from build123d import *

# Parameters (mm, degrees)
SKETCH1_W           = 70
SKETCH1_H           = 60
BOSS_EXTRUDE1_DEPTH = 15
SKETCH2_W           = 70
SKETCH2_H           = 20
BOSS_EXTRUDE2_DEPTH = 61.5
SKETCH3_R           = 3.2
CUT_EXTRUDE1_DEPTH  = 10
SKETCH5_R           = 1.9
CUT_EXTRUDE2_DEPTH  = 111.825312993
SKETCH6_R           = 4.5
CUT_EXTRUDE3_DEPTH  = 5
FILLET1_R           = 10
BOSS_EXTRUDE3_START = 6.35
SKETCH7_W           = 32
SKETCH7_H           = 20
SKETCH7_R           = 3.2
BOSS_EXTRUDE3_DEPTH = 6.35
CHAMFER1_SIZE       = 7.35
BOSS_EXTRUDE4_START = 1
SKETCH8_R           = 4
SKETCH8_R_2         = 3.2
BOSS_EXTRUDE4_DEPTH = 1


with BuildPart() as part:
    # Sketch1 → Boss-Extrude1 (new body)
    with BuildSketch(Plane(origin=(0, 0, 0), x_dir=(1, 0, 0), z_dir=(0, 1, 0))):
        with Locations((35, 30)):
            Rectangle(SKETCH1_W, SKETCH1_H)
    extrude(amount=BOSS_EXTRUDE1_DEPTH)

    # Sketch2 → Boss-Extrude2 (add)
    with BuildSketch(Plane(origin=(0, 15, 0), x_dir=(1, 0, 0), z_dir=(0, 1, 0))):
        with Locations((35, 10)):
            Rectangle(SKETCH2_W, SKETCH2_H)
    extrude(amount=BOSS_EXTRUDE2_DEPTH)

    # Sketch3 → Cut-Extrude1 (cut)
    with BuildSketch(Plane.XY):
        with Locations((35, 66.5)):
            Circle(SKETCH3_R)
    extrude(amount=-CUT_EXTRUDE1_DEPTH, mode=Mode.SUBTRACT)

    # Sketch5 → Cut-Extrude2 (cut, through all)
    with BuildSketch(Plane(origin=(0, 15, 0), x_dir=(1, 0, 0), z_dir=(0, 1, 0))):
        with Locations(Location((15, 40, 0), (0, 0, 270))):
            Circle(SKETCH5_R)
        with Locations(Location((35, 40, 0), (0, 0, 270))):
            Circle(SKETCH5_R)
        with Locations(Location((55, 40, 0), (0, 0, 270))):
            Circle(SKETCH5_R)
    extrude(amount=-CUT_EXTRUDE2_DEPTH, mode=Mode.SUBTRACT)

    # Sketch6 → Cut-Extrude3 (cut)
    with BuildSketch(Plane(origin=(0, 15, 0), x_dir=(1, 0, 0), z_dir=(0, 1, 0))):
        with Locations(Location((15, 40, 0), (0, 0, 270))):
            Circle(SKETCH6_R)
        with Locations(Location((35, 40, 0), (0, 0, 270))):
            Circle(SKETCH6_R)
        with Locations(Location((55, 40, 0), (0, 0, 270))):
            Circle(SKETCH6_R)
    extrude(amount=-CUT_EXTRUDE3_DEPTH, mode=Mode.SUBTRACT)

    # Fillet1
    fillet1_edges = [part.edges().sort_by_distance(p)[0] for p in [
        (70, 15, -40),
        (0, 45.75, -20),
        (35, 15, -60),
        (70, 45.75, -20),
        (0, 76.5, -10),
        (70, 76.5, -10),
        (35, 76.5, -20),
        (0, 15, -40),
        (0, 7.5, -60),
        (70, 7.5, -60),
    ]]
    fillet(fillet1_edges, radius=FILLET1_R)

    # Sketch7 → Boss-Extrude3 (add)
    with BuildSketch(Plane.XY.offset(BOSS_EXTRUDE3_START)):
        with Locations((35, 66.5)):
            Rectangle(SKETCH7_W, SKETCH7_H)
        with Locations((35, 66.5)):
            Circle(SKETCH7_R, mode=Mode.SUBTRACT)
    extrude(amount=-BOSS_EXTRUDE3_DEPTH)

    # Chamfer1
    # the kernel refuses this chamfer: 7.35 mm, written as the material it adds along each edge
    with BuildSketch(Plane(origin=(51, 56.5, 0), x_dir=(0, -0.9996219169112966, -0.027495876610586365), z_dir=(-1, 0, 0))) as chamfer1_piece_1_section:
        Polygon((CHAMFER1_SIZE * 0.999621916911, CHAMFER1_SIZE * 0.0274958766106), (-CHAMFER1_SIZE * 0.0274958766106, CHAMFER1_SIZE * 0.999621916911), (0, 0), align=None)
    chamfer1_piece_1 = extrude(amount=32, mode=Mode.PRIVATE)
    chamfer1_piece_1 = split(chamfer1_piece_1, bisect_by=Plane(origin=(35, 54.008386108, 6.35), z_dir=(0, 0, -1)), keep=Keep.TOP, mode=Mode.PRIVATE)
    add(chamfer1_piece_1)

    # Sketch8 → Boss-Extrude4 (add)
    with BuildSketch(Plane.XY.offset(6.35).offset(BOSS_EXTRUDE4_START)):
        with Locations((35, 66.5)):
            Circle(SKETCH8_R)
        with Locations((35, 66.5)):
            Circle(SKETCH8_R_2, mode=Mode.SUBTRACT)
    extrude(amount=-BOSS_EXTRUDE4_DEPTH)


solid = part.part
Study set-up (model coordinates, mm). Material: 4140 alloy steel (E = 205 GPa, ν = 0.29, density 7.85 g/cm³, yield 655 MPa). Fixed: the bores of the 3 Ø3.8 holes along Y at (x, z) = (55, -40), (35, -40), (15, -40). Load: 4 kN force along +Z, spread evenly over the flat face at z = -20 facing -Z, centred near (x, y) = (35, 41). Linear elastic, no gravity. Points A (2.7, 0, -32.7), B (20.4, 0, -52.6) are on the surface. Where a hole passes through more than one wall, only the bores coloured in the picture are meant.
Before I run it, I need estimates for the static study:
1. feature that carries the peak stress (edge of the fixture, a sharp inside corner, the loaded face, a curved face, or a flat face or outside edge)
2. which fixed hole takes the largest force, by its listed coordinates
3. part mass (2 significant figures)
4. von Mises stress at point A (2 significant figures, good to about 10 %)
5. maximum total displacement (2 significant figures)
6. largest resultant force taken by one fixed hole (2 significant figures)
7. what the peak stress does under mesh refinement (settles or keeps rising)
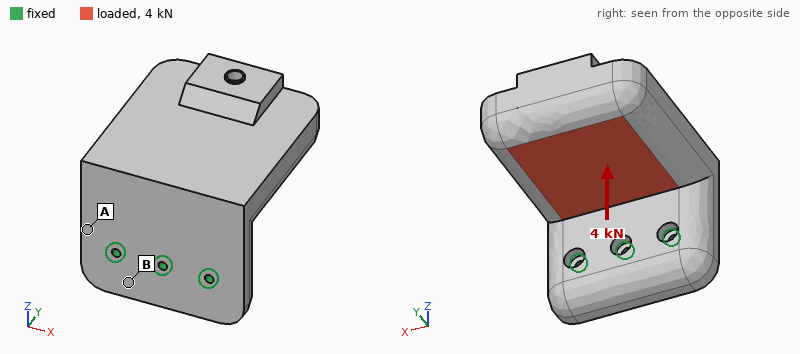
edge of the fixture
(35, -40)
1.1 kg
45 MPa
0.13 mm
1.6 kN
keeps rising
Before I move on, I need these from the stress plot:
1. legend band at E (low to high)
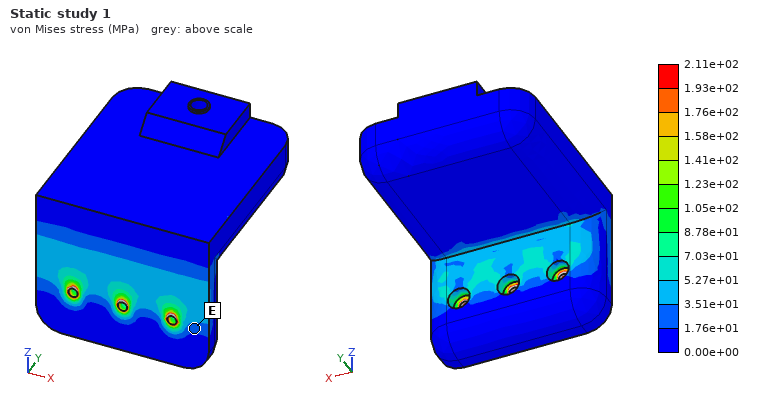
1.76e+01 to 3.51e+01 MPa
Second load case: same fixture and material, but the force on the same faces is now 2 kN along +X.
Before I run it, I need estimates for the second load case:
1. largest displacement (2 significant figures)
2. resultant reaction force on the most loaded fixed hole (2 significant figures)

17 µm
1.9 kN
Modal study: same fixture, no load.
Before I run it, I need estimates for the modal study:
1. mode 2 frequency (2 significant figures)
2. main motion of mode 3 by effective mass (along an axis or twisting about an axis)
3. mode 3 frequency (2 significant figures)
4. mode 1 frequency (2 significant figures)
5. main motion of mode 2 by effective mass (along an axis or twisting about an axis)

2300 Hz
along Y
4700 Hz
1100 Hz
along X
